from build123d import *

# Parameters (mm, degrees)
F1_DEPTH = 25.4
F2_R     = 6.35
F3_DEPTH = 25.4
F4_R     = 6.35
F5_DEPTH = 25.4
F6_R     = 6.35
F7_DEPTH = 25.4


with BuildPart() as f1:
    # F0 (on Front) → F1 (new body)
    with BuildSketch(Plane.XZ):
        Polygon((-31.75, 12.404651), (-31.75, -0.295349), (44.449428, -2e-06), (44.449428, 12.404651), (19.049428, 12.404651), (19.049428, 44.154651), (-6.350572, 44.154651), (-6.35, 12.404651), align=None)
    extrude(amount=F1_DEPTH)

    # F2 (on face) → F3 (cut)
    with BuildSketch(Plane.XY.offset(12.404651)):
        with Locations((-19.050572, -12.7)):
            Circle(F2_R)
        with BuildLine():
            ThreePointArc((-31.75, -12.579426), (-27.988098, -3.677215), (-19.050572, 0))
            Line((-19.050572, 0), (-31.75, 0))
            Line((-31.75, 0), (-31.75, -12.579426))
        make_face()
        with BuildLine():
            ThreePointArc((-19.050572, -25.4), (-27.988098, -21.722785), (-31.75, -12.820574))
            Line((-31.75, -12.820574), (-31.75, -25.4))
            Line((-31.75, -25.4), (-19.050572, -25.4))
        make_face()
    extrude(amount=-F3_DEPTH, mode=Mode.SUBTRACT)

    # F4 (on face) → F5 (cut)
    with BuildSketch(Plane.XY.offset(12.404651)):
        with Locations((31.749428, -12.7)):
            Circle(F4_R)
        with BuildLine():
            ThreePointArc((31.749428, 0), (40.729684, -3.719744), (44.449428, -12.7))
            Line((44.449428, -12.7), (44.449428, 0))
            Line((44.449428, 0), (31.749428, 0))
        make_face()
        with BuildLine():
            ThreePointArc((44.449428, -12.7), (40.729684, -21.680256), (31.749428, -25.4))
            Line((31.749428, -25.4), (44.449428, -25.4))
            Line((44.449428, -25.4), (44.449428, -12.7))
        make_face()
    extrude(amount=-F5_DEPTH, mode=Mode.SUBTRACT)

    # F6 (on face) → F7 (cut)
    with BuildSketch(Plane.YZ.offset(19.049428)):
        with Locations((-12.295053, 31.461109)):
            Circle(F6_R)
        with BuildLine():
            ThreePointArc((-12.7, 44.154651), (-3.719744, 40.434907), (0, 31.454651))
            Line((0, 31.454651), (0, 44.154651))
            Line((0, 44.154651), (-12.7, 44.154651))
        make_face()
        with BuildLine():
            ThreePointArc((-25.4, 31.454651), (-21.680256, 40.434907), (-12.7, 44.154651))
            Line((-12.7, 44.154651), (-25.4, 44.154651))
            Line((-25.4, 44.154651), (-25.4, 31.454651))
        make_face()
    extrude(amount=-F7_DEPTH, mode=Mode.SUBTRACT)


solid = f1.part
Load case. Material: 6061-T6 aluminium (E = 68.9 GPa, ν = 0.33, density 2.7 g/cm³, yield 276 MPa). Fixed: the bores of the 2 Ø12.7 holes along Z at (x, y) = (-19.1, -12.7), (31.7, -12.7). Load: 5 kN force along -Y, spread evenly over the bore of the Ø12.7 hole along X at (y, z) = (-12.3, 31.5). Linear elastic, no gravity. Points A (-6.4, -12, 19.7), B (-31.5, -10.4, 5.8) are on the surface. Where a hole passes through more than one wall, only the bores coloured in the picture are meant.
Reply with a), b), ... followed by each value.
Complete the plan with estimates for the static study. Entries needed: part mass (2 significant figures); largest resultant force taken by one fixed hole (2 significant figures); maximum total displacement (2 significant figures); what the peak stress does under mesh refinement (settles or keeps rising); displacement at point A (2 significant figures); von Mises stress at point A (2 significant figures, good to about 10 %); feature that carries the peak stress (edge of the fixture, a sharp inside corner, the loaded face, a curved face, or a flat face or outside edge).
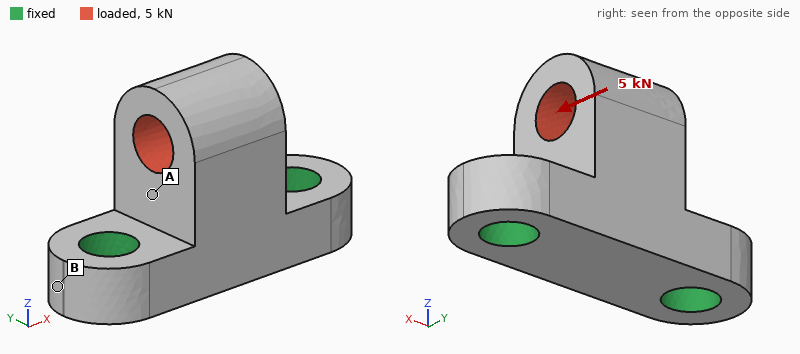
a) 94 g
b) 2.5 kN
c) 0.11 mm
d) keeps rising
e) 0.038 mm
f) 39 MPa
g) edge of the fixture
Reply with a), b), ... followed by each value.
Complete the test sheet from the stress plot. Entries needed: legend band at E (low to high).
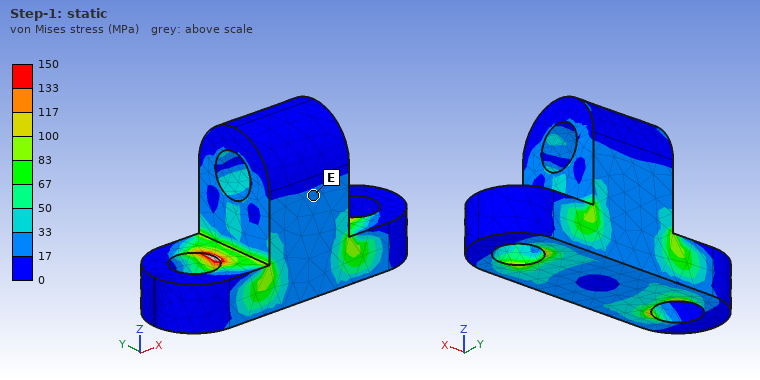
a) 17 to 33 MPa
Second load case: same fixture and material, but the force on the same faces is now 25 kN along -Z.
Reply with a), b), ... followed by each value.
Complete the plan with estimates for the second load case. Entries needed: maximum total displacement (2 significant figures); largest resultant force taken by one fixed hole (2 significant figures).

a) 59 µm
b) 13 kN
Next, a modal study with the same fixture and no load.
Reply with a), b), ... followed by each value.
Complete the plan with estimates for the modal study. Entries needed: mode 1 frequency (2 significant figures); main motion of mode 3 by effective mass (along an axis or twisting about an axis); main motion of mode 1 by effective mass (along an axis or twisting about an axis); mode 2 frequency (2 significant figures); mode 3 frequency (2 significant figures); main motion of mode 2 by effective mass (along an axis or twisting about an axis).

a) 6900 Hz
b) along Z
c) along Y
d) 12 kHz
e) 17 kHz
f) along X
